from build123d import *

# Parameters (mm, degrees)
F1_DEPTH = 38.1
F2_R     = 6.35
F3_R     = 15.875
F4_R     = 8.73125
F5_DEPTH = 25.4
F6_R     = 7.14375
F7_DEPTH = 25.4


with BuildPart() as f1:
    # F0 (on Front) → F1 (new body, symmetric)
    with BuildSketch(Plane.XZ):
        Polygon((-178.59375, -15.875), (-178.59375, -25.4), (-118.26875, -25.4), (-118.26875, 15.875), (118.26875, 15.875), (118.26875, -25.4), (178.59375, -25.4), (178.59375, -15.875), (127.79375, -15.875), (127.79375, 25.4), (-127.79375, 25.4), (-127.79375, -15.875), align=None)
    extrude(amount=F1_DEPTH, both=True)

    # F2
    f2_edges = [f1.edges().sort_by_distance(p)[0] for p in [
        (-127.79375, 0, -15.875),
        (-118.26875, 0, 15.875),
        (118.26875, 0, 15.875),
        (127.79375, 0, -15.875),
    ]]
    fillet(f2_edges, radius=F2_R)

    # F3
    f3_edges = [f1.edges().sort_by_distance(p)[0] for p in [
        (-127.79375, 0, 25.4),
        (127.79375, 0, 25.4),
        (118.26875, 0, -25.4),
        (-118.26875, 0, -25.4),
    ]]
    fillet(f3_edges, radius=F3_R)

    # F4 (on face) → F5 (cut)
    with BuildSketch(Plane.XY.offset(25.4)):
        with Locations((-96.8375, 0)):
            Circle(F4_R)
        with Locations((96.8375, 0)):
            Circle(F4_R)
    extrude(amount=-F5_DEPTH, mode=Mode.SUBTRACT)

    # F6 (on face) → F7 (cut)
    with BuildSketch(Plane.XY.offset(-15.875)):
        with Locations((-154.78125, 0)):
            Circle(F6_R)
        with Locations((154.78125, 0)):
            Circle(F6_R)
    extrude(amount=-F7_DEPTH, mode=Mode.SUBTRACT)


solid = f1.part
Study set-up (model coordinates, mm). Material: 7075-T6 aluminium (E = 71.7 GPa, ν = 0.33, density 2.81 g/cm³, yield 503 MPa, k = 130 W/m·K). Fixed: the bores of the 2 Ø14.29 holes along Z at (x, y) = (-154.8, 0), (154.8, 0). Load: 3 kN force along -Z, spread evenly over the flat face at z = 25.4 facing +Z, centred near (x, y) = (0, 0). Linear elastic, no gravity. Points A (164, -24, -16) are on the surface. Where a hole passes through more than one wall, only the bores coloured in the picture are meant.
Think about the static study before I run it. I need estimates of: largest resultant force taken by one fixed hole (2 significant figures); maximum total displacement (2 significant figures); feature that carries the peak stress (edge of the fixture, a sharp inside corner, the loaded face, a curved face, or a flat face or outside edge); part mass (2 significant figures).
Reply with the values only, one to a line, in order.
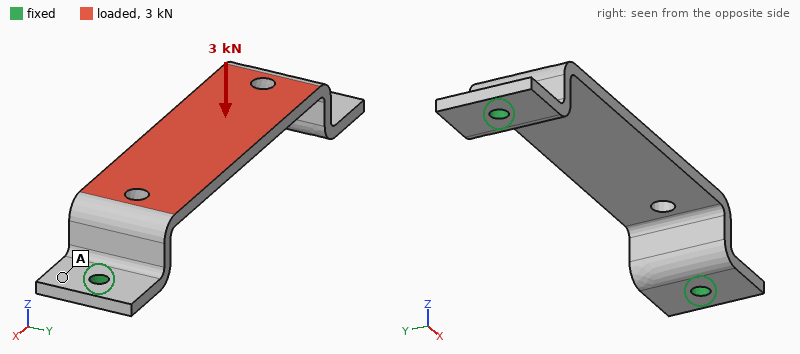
2.7 kN
0.42 mm
a curved face
840 g
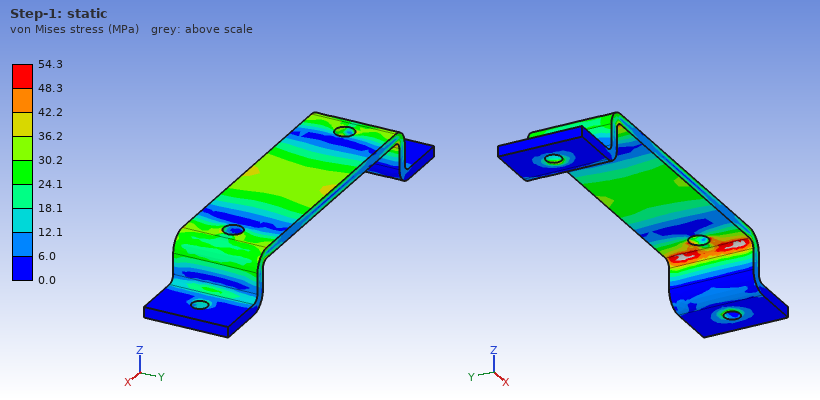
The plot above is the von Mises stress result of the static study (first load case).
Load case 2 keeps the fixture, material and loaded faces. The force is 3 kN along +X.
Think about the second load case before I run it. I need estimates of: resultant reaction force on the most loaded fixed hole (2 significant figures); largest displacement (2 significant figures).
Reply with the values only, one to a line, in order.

1.5 kN
0.15 mm
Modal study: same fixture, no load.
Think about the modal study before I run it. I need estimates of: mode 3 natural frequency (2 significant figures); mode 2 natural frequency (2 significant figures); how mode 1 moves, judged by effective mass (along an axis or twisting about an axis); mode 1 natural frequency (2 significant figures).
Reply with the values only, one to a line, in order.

950 Hz
930 Hz
along Z
730 Hz
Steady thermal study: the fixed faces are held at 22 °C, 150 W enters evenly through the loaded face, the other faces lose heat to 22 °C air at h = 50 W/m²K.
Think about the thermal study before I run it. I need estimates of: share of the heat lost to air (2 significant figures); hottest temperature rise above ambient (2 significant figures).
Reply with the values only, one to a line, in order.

53 %
63 K
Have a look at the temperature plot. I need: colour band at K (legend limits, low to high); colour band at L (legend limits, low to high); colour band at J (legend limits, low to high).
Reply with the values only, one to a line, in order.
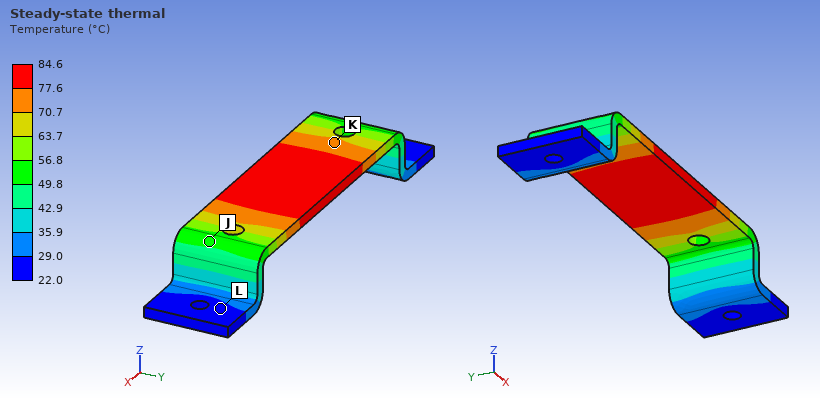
70.7 to 77.6 °C
22.0 to 29.0 °C
49.8 to 56.8 °C
